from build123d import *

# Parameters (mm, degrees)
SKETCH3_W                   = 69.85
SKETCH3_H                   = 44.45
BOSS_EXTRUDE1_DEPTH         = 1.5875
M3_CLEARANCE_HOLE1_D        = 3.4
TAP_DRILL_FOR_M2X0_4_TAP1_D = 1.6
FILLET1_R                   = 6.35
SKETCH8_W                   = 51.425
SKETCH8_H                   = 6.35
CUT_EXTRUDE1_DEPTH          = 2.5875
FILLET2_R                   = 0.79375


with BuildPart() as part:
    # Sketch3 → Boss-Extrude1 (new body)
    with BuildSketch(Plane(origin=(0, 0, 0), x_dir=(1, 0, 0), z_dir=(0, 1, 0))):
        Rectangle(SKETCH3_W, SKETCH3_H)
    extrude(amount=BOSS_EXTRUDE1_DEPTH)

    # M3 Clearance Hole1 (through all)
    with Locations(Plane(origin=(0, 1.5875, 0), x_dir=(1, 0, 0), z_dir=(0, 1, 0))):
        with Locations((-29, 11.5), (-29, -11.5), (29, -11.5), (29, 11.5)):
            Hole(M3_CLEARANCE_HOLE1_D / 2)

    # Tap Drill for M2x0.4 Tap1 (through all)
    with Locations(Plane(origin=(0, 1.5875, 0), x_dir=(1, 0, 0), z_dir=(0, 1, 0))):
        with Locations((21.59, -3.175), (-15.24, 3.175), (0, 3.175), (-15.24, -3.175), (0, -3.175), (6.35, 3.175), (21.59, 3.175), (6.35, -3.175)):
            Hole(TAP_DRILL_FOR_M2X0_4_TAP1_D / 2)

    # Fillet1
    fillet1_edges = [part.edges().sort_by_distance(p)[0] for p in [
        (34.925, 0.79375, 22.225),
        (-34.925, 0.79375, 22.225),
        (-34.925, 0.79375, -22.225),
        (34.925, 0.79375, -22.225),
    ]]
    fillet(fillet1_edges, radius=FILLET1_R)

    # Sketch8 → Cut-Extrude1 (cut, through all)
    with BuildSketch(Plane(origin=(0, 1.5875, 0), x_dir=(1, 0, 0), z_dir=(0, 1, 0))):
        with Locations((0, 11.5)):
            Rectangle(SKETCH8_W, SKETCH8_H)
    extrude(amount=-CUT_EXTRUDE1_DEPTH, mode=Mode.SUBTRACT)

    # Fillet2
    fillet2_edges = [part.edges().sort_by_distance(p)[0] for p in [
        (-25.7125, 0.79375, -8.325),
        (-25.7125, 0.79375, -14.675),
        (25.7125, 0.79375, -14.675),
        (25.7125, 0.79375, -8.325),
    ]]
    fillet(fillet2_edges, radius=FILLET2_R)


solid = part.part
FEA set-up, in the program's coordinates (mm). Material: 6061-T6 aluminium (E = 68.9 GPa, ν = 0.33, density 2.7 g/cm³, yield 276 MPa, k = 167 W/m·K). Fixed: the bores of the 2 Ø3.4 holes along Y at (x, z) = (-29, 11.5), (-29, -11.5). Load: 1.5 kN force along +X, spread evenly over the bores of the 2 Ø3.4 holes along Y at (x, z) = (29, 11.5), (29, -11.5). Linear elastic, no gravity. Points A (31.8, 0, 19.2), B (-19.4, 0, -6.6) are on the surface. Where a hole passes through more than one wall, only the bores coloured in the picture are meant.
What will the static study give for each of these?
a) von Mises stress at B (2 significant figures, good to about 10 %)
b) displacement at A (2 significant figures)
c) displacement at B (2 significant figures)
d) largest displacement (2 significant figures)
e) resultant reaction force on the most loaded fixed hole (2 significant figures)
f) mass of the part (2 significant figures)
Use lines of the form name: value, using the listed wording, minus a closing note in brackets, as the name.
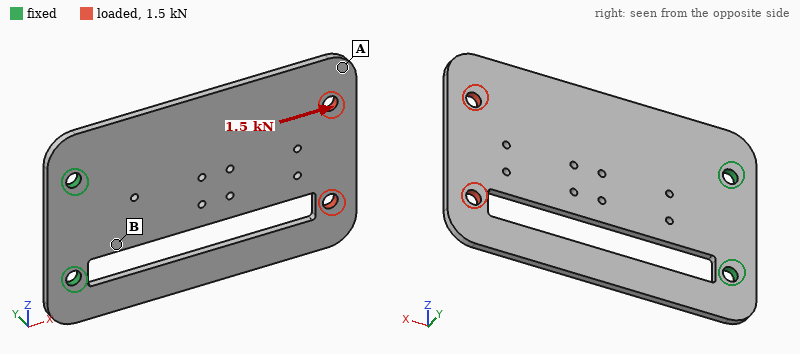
von Mises stress at B: 36 MPa
displacement at A: 27 µm
displacement at B: 8.8 µm
largest displacement: 50 µm
resultant reaction force on the most loaded fixed hole: 790 N
mass of the part: 12 g
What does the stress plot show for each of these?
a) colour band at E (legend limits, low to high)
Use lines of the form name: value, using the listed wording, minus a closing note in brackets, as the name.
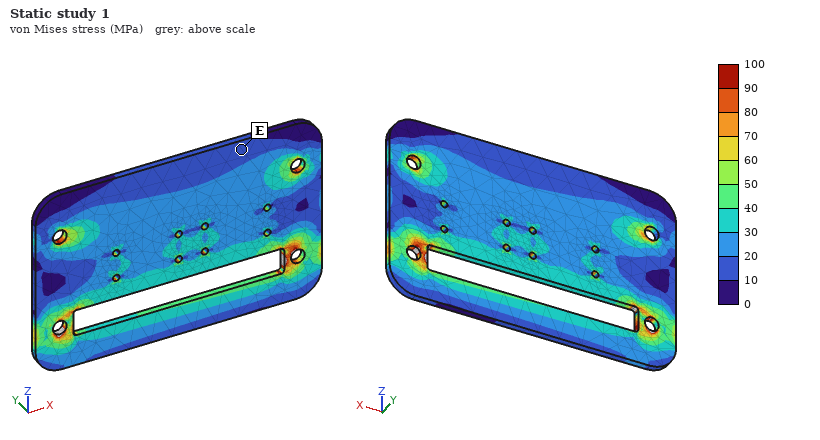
colour band at E: 10 to 20 MPa
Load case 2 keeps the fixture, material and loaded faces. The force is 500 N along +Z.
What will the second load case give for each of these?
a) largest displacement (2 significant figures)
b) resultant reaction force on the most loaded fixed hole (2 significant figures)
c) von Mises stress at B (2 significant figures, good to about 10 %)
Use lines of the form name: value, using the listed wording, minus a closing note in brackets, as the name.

largest displacement: 0.19 mm
resultant reaction force on the most loaded fixed hole: 1.2 kN
von Mises stress at B: 82 MPa
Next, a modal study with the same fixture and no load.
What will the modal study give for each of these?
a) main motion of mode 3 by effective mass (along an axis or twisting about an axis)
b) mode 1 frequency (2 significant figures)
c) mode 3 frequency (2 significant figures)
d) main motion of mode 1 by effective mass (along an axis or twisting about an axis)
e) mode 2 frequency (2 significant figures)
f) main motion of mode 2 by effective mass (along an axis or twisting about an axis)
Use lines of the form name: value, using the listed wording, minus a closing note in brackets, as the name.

main motion of mode 3 by effective mass: along Y
mode 1 frequency: 310 Hz
mode 3 frequency: 1900 Hz
main motion of mode 1 by effective mass: along Y
mode 2 frequency: 970 Hz
main motion of mode 2 by effective mass: twisting about X
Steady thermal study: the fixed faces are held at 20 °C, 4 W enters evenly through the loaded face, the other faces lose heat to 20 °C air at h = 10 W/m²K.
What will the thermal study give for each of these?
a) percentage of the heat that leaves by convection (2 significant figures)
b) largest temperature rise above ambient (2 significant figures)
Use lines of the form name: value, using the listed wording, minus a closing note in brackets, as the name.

percentage of the heat that leaves by convection: 16 %
largest temperature rise above ambient: 24 K
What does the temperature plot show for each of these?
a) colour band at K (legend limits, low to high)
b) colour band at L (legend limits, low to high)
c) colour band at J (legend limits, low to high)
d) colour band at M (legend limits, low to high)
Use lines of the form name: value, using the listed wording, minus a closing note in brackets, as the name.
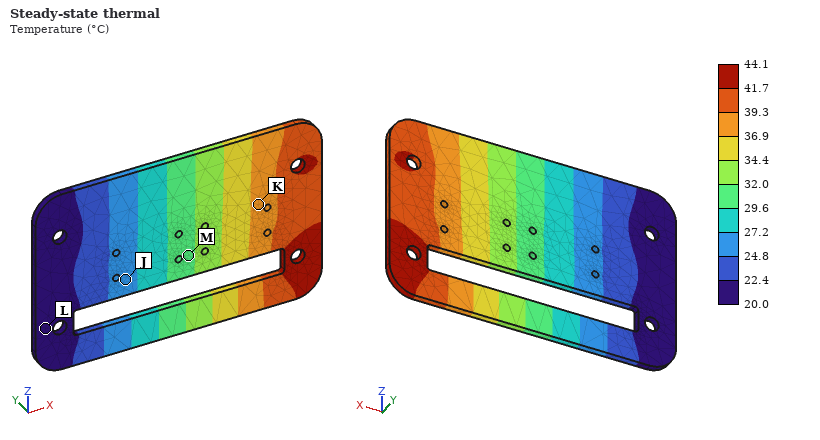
colour band at K: 36.9 to 39.3 °C
colour band at L: 20.0 to 22.4 °C
colour band at J: 24.8 to 27.2 °C
colour band at M: 29.6 to 32.0 °C
